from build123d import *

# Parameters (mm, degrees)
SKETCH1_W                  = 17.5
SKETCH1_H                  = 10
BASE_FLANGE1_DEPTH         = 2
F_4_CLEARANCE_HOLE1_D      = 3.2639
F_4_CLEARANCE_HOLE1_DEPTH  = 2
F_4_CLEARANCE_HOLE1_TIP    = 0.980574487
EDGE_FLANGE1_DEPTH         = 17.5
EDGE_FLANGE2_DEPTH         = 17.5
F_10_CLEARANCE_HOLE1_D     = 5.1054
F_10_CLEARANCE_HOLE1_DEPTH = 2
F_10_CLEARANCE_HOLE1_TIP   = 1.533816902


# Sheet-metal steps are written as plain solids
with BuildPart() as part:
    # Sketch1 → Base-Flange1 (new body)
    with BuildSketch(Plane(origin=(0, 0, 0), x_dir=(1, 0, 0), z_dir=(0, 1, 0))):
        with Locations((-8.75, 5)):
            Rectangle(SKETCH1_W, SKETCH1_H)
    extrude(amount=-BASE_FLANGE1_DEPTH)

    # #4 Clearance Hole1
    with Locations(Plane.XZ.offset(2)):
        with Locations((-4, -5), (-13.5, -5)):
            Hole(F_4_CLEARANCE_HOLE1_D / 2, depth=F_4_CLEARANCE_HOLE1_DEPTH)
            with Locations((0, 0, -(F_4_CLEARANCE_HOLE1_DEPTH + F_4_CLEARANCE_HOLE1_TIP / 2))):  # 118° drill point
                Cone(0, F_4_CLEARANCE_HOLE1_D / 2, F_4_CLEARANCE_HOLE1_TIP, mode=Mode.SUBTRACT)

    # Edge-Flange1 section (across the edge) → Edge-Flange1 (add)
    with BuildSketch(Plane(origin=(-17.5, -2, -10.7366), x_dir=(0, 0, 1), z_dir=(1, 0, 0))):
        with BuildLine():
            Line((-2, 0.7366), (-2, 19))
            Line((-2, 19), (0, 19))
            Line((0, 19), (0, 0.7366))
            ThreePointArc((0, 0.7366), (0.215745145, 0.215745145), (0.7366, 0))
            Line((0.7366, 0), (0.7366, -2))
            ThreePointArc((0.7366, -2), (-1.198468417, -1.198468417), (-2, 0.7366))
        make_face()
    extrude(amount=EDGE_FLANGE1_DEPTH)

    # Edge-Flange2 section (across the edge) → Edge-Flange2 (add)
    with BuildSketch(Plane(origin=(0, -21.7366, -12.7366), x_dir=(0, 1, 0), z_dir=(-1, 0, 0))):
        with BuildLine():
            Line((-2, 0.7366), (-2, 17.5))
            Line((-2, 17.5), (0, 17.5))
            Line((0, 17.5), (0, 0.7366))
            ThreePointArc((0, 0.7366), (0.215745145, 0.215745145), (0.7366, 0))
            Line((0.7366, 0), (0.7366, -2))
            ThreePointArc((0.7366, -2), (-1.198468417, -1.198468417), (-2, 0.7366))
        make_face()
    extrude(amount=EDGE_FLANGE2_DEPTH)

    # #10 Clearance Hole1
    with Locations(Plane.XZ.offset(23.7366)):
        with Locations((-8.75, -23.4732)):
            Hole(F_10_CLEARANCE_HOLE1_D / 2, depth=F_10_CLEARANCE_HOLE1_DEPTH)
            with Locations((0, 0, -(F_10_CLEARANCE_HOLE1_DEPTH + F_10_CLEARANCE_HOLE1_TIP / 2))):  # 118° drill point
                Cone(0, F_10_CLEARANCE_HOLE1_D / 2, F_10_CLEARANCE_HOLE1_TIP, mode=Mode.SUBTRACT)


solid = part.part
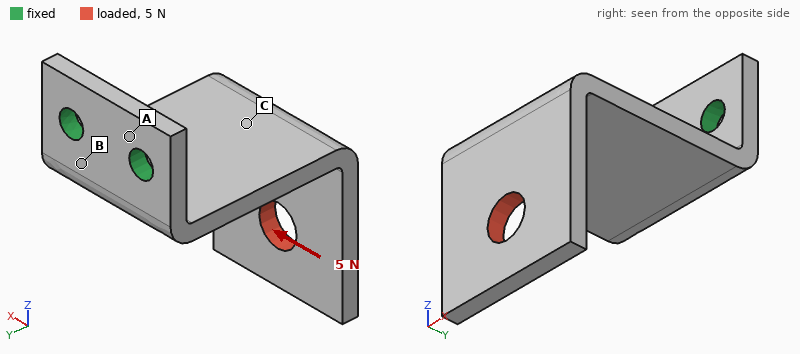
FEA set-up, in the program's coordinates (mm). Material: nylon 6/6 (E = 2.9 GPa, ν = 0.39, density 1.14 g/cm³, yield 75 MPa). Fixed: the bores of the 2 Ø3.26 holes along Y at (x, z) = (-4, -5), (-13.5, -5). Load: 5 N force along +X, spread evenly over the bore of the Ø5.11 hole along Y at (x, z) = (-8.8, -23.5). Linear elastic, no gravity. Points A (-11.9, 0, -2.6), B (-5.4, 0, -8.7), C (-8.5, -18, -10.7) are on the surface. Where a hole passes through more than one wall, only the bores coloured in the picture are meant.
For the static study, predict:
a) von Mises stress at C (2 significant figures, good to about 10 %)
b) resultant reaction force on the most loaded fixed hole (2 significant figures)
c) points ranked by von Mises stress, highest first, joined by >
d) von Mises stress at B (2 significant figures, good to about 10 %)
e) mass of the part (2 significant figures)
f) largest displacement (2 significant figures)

3.4 MPa
12 N
C > B > A
1.1 MPa
1.9 g
0.43 mm
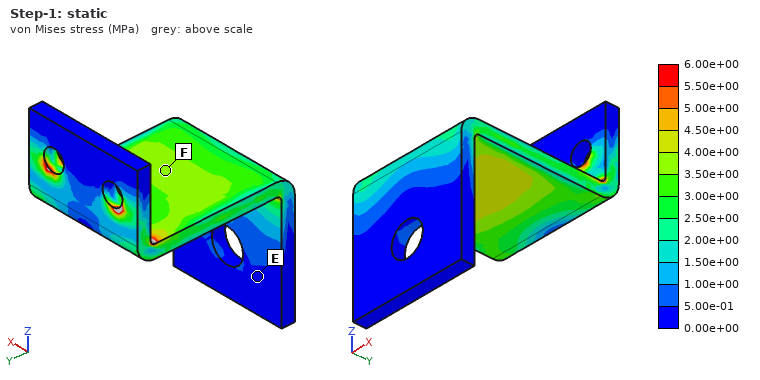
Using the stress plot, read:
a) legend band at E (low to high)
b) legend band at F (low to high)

0.00e+00 to 5.00e-01 MPa
3.50e+00 to 4.00e+00 MPa
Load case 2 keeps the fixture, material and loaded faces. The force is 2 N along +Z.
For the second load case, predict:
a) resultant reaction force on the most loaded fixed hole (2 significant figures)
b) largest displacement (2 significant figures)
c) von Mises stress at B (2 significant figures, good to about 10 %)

1.3 N
0.50 mm
3.4 MPa
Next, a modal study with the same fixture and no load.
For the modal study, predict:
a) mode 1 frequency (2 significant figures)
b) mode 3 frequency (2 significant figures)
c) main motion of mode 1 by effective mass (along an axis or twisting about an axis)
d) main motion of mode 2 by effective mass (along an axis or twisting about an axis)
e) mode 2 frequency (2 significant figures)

360 Hz
1300 Hz
along Z
along X
820 Hz
